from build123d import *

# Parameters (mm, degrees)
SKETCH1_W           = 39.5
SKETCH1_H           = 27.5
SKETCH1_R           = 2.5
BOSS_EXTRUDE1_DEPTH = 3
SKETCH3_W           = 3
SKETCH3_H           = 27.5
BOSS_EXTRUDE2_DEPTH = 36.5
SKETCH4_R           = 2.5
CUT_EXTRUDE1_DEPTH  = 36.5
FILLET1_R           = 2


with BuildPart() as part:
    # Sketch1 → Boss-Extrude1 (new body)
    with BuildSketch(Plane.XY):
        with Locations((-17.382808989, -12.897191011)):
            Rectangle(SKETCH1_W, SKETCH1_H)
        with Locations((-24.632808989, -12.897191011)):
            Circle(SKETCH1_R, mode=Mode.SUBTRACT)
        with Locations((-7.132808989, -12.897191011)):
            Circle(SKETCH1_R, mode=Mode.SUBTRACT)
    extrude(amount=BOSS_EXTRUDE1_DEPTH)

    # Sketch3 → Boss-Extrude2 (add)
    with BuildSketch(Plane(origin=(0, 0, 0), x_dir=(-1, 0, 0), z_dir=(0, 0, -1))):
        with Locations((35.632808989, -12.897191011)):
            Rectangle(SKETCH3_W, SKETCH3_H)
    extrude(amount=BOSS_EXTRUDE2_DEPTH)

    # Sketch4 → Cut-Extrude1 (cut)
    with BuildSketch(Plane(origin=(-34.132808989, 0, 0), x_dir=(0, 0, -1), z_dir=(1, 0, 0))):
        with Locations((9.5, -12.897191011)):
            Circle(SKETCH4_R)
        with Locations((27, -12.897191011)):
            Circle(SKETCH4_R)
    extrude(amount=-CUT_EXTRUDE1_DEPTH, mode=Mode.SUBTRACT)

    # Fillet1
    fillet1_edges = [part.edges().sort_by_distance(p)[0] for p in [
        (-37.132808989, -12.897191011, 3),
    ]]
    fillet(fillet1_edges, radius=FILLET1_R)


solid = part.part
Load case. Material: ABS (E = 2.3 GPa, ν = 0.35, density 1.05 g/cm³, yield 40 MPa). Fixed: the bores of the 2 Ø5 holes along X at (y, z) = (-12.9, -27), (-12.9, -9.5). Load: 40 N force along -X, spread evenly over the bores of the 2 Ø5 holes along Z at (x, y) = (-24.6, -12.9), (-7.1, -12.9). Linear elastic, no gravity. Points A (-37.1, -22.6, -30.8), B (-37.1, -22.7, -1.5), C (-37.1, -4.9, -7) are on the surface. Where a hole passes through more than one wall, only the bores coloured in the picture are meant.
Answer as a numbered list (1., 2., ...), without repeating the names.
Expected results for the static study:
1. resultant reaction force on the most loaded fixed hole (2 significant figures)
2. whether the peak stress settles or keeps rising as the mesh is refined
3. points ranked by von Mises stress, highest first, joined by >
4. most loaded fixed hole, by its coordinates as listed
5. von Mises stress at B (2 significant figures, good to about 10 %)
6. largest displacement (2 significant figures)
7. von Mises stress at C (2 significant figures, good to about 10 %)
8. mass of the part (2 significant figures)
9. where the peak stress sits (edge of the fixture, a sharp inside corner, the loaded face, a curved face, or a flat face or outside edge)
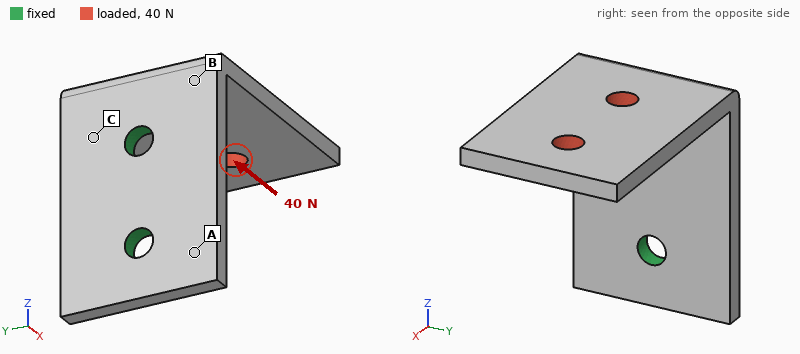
1. 46 N
2. keeps rising
3. C > B > A
4. (-12.9, -9.5)
5. 2.5 MPa
6. 0.61 mm
7. 4.4 MPa
8. 6.3 g
9. edge of the fixture
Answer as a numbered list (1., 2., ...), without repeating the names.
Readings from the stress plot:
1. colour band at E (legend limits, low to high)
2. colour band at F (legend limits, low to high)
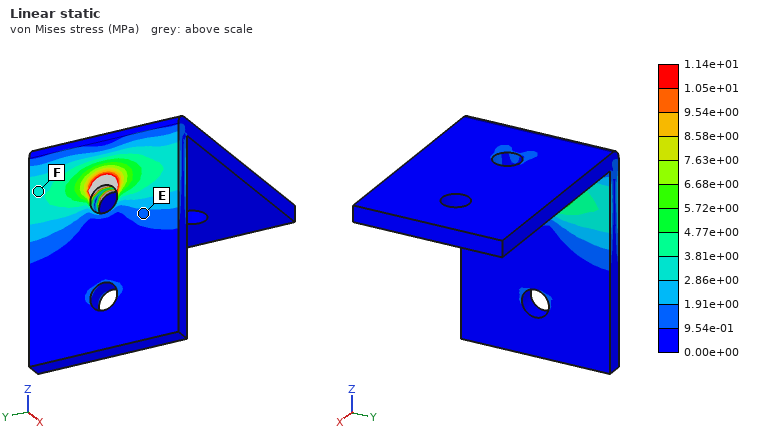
1. 9.54e-01 to 1.91e+00 MPa
2. 2.86e+00 to 3.81e+00 MPa
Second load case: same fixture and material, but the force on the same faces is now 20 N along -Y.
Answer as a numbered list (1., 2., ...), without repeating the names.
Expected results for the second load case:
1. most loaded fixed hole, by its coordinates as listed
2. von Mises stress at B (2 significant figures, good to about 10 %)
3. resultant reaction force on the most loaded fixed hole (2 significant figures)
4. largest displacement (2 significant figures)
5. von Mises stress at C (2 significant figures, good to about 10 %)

1. (-12.9, -9.5)
2. 2.7 MPa
3. 28 N
4. 0.63 mm
5. 3.8 MPa
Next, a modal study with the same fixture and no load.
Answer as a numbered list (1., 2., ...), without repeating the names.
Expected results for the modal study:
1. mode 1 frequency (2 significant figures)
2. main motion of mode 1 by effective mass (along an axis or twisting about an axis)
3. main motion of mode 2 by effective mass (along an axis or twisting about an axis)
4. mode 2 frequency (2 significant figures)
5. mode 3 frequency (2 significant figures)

1. 350 Hz
2. along Z
3. along Y
4. 610 Hz
5. 1400 Hz
